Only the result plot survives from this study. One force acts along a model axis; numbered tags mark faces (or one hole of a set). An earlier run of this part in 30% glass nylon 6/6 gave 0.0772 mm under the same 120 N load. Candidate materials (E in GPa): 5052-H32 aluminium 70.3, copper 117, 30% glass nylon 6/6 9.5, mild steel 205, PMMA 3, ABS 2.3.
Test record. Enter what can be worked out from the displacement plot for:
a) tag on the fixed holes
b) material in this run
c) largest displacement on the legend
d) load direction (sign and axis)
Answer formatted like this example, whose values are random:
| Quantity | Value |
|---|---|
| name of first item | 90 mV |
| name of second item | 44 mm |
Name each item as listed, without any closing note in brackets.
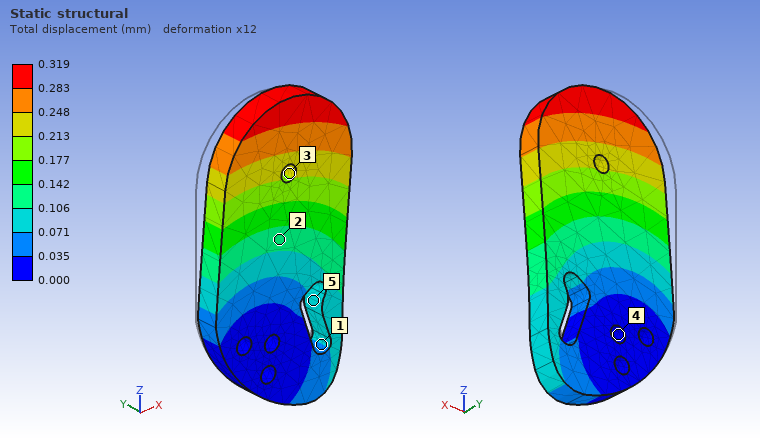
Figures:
| Quantity | Value |
|---|---|
| tag on the fixed holes | 4 |
| material in this run | ABS |
| largest displacement on the legend | 0.319 mm |
| load direction | +X |
